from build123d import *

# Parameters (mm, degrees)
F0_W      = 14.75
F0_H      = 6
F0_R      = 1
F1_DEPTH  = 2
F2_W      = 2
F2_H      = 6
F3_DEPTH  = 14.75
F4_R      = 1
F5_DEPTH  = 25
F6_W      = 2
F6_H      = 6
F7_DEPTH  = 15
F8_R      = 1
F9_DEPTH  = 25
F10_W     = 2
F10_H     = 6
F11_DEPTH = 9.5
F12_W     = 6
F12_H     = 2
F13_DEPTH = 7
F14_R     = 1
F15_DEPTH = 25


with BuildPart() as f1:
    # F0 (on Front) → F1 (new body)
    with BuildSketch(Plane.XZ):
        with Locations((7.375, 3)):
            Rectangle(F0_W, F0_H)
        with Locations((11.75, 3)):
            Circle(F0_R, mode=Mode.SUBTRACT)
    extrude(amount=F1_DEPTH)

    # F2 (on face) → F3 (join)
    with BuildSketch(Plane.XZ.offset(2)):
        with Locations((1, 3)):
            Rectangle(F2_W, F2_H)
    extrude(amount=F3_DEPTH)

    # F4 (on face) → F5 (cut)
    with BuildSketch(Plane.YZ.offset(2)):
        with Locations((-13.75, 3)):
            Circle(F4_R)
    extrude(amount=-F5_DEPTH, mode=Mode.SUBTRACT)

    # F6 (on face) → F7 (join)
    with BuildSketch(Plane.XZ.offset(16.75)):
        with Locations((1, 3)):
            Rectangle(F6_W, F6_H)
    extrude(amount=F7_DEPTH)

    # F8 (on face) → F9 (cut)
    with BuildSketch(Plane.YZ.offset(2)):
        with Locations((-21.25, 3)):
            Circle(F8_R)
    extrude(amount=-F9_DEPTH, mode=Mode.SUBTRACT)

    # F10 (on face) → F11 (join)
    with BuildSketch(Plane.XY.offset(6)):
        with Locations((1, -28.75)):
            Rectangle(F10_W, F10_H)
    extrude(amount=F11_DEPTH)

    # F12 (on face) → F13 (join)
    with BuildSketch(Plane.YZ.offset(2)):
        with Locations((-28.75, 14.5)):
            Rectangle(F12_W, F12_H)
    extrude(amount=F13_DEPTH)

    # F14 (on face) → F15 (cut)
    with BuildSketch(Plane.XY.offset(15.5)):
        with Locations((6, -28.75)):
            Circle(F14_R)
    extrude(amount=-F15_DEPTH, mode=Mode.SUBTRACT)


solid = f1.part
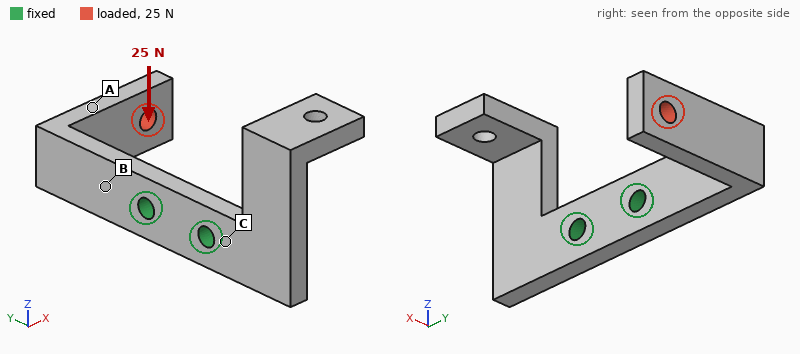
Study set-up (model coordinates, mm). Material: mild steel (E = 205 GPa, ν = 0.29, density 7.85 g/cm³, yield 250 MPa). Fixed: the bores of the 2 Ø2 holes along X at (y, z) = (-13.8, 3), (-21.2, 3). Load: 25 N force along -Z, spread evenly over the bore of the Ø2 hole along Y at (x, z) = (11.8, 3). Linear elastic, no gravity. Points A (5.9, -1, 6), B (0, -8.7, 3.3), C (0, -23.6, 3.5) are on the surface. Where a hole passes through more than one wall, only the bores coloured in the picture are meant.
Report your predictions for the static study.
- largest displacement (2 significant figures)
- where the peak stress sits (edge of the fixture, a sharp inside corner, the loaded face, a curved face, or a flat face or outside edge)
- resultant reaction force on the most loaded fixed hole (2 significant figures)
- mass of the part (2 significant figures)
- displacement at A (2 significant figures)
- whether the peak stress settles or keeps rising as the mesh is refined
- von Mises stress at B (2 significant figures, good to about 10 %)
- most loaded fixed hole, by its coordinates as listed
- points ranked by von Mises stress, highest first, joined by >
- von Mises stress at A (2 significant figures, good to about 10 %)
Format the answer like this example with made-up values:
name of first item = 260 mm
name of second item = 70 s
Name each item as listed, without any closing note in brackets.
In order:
largest displacement = 47 µm
where the peak stress sits = edge of the fixture
resultant reaction force on the most loaded fixed hole = 44 N
mass of the part = 5.5 g
displacement at A = 20 µm
whether the peak stress settles or keeps rising as the mesh is refined = keeps rising
von Mises stress at B = 64 MPa
most loaded fixed hole, by its coordinates as listed = (-13.8, 3)
points ranked by von Mises stress, highest first, joined by > = B > A > C
von Mises stress at A = 12 MPa
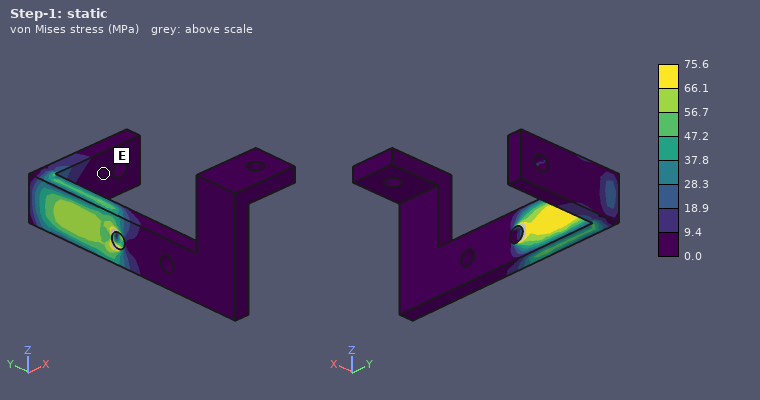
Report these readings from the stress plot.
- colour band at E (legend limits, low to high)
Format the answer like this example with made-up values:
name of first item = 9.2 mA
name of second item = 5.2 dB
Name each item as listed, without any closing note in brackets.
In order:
colour band at E = 0.0 to 9.4 MPa
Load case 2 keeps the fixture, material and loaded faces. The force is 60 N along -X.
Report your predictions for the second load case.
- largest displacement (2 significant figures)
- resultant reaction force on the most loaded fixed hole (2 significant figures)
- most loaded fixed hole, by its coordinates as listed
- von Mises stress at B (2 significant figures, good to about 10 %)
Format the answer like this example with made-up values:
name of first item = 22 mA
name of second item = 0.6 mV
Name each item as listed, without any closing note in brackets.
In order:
largest displacement = 92 µm
resultant reaction force on the most loaded fixed hole = 71 N
most loaded fixed hole, by its coordinates as listed = (-13.8, 3)
von Mises stress at B = 110 MPa
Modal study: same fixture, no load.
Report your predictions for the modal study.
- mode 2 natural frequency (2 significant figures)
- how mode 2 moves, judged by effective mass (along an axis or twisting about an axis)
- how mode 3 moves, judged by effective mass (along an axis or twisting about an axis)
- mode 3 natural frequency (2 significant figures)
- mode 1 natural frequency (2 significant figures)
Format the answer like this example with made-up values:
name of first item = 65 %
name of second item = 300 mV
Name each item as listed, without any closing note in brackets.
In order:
mode 2 natural frequency = 4000 Hz
how mode 2 moves, judged by effective mass = along X
how mode 3 moves, judged by effective mass = along Z
mode 3 natural frequency = 4900 Hz
mode 1 natural frequency = 3300 Hz
